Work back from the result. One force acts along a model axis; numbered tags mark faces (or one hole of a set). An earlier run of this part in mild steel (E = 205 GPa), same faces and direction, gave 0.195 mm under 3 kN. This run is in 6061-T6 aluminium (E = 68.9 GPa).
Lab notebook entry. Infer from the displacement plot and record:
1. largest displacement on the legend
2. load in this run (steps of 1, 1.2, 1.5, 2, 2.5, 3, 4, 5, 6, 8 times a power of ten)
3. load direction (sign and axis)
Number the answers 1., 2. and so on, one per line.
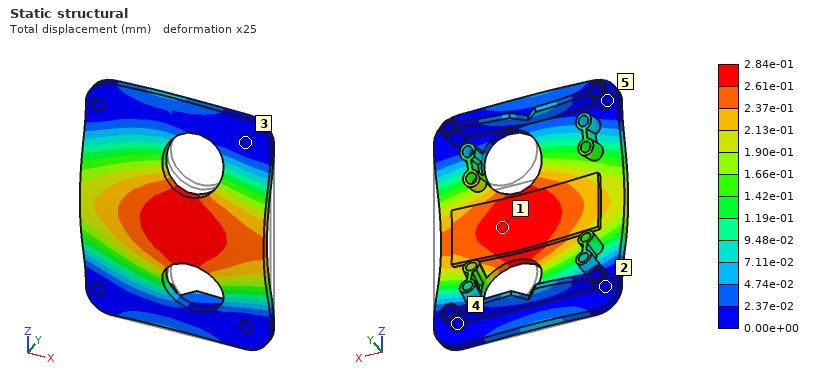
1. 2.84e-01 mm
2. 1.5 kN
3. -Y
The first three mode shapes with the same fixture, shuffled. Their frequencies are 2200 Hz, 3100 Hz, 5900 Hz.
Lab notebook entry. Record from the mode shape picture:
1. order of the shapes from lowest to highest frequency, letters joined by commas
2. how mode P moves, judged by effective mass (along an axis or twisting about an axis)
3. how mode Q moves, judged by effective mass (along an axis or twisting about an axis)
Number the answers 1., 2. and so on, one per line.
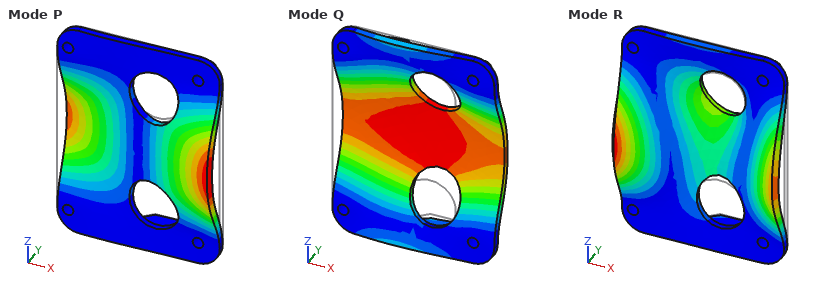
1. Q, P, R
2. twisting about Z
3. along Y
